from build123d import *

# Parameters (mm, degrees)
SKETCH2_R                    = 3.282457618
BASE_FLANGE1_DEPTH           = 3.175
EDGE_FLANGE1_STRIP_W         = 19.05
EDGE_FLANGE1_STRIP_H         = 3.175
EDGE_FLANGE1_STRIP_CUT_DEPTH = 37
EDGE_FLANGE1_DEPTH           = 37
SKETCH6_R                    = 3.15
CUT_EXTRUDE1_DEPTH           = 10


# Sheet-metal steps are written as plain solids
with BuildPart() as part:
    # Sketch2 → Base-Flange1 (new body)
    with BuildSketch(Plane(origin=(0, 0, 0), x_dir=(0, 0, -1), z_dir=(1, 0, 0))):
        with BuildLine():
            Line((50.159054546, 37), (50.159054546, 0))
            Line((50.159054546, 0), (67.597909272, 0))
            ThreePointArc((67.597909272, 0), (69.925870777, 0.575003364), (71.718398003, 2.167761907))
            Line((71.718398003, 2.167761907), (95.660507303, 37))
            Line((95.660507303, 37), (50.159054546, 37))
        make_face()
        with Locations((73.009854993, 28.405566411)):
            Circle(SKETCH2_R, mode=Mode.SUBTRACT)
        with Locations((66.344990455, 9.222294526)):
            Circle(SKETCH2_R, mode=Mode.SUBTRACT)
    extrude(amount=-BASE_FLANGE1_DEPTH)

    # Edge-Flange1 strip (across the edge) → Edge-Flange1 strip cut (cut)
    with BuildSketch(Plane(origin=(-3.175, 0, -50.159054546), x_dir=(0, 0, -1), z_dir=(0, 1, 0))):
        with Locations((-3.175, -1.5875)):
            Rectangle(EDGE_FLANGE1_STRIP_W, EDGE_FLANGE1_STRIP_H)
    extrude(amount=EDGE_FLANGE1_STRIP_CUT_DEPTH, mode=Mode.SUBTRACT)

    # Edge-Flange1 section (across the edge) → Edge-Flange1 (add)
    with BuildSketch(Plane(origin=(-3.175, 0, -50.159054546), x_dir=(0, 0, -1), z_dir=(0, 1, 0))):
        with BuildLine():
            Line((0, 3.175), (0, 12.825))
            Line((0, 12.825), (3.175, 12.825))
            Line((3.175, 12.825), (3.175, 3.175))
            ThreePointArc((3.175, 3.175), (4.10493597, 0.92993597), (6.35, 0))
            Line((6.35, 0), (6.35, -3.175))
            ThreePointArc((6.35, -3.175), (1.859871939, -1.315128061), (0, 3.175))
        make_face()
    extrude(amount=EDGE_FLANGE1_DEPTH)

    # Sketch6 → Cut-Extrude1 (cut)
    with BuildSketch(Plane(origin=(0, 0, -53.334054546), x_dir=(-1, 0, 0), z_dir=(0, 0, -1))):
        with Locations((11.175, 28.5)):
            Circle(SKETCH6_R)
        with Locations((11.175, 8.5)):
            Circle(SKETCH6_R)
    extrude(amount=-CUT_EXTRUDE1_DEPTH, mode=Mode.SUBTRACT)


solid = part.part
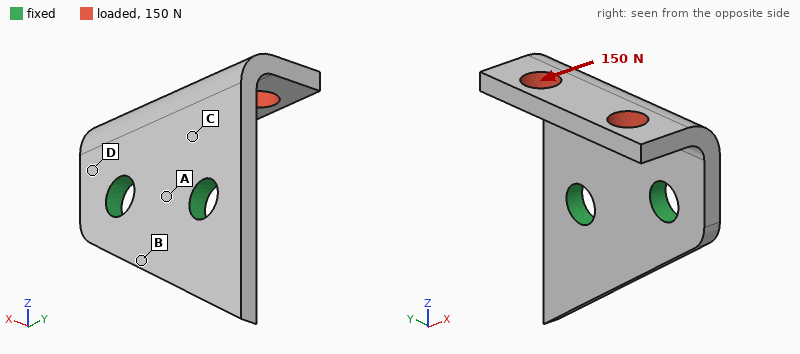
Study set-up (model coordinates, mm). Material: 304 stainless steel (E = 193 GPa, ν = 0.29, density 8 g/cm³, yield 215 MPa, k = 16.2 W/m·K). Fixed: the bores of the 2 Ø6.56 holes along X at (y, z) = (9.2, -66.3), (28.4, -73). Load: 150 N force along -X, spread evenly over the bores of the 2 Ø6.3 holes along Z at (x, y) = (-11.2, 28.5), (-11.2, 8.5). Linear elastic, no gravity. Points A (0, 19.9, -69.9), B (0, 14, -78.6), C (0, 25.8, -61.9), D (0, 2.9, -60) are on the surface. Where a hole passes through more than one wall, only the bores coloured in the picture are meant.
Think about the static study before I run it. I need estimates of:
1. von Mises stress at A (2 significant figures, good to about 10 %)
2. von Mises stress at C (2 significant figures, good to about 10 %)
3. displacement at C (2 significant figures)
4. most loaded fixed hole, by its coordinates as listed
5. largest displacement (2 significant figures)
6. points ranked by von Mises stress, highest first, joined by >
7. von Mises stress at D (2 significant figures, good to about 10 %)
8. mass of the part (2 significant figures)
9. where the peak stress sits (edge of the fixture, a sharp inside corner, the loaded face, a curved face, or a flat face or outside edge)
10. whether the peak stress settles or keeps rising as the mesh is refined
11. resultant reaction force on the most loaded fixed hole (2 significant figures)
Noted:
9.6 MPa
16 MPa
3.1 µm
(9.2, -66.3)
20 µm
D > C > A > B
21 MPa
38 g
edge of the fixture
keeps rising
110 N
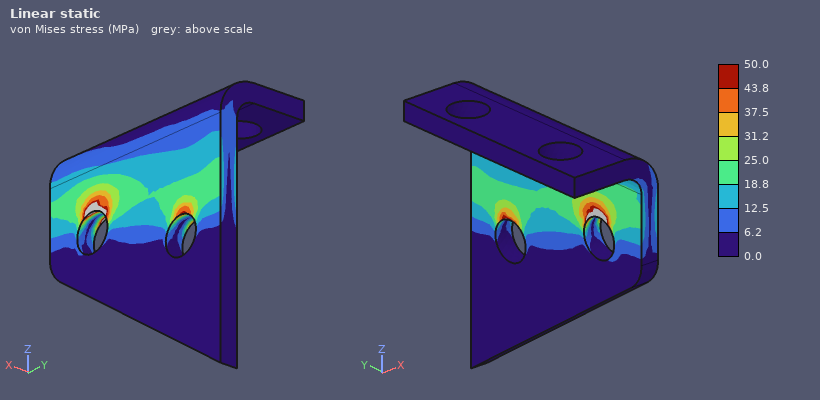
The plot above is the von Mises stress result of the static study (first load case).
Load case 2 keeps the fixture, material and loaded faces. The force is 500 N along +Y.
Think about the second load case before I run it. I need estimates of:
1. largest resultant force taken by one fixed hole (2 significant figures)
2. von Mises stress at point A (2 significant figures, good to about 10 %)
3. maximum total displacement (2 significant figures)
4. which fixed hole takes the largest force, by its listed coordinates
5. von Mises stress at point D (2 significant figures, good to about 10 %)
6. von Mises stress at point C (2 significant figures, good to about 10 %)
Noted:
510 N
13 MPa
37 µm
(9.2, -66.3)
29 MPa
27 MPa
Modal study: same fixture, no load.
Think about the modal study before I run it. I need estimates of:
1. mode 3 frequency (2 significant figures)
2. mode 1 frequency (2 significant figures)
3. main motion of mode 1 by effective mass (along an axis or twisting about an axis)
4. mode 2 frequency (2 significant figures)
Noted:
9500 Hz
4200 Hz
along X
6700 Hz
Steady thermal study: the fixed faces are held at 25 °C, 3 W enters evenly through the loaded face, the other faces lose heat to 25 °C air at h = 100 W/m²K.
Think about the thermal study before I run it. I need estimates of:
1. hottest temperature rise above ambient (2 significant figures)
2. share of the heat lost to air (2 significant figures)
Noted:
22 K
68 %
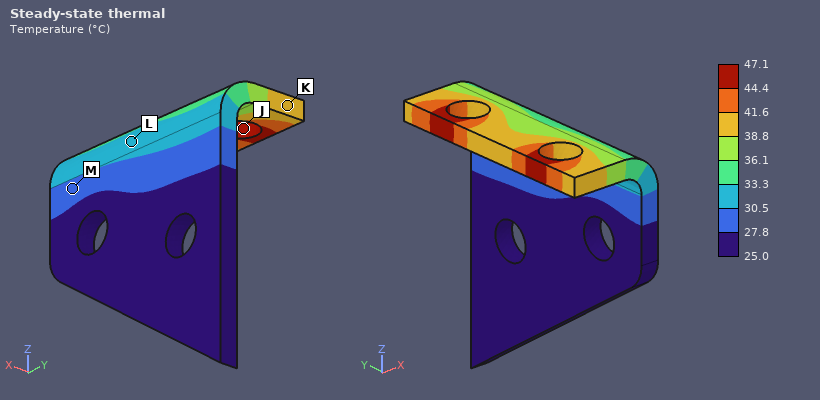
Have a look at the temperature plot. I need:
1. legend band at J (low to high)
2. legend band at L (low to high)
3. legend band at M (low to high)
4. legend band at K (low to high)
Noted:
44.4 to 47.1 °C
30.5 to 33.3 °C
27.8 to 30.5 °C
38.8 to 41.6 °C
